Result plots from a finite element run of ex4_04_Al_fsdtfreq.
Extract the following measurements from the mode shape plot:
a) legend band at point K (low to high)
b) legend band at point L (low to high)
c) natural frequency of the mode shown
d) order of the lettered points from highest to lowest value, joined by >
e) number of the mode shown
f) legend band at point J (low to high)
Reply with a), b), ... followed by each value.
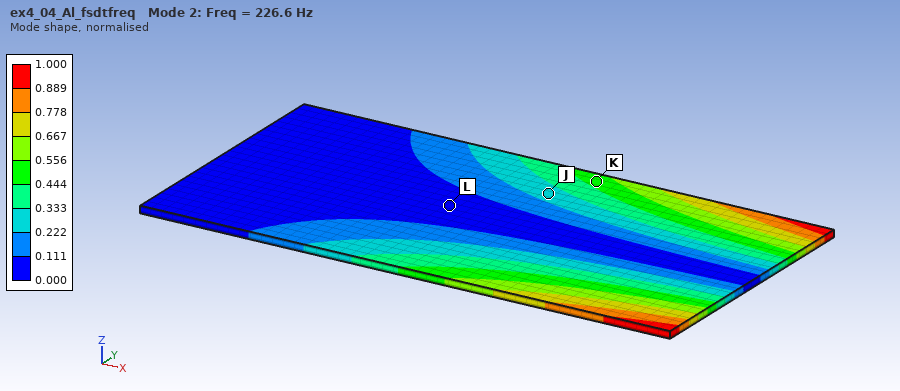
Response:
a) 0.444 to 0.556
b) 0.000 to 0.111
c) 226.6 Hz
d) K > J > L
e) 2
f) 0.222 to 0.333
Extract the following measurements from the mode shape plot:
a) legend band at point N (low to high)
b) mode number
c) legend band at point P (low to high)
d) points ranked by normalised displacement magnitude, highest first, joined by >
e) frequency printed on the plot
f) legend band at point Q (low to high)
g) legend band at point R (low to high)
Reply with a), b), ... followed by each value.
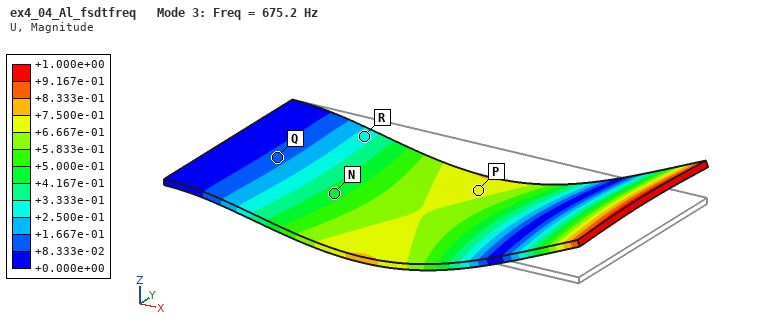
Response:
a) +4.167e-01 to +5.000e-01
b) 3
c) +6.667e-01 to +7.500e-01
d) P > N > R > Q
e) 675.2 Hz
f) +8.333e-02 to +1.667e-01
g) +2.500e-01 to +3.333e-01
